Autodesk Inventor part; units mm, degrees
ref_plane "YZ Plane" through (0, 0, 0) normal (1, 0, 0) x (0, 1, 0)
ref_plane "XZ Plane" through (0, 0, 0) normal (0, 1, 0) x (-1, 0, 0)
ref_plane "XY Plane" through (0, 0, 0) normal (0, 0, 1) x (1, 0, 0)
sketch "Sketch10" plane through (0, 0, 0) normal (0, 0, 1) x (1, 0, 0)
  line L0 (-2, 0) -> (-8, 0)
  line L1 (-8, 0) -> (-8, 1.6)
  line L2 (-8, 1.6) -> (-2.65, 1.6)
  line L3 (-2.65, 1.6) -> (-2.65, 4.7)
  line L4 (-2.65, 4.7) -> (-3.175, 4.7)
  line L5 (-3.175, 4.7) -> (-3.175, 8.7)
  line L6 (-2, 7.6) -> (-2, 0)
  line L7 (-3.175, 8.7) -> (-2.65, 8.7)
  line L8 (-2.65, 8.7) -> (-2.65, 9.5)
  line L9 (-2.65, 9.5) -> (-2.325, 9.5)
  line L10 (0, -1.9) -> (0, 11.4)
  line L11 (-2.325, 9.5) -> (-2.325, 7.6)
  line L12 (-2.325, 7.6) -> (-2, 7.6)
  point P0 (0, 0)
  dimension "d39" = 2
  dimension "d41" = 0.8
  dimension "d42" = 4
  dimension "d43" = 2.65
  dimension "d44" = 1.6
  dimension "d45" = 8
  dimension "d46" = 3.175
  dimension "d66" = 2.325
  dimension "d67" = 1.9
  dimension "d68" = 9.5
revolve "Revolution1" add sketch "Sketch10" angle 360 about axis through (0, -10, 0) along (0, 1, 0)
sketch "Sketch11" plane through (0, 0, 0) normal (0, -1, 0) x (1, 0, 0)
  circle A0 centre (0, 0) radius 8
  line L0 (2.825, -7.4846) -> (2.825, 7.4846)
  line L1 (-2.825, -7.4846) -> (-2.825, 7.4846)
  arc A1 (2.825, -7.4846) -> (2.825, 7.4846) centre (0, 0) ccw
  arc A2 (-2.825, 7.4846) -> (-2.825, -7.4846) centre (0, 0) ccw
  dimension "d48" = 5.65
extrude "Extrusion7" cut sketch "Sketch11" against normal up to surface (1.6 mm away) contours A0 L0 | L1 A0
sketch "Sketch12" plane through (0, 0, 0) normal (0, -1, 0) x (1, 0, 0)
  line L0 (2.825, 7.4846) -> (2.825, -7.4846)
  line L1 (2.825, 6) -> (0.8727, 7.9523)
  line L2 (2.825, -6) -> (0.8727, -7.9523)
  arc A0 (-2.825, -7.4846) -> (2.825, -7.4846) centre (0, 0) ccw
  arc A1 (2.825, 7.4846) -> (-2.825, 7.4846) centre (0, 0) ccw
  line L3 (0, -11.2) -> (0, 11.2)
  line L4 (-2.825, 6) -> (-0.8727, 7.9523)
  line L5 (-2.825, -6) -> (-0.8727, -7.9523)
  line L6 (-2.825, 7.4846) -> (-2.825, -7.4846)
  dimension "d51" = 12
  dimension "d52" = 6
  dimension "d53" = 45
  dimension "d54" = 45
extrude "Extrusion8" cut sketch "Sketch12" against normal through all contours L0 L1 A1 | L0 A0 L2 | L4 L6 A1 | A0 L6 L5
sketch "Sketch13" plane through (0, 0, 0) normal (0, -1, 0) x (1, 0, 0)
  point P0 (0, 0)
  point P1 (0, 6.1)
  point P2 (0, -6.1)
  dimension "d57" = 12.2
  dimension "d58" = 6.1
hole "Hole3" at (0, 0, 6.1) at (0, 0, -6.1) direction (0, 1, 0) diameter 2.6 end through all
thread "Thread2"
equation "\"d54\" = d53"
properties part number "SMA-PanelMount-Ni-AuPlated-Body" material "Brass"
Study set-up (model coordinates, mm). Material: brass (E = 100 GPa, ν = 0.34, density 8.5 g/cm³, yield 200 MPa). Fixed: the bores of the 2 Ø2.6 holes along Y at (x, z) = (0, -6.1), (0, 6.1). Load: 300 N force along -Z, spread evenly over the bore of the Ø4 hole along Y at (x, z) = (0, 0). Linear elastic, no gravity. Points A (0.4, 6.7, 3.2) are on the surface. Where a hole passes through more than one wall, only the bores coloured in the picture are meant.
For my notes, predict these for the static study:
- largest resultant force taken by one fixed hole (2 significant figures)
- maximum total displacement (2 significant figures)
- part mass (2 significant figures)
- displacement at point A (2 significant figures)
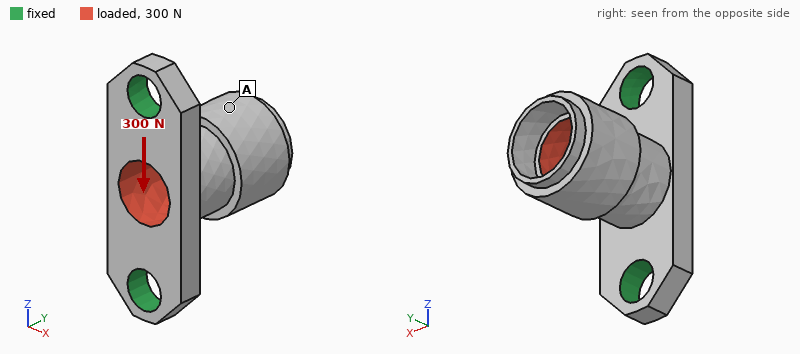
190 N
18 µm
1.7 g
14 µm
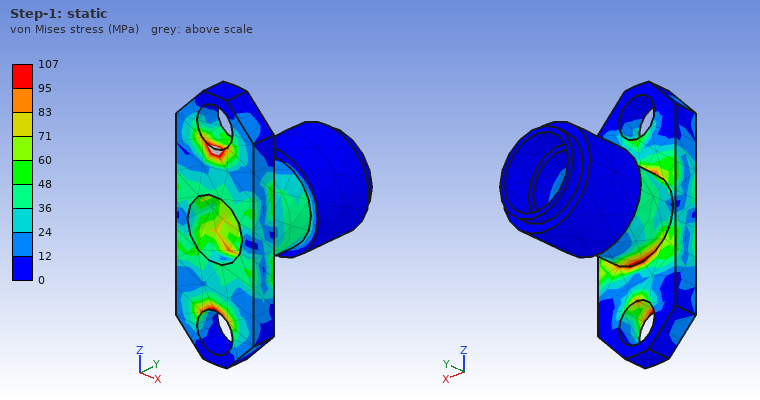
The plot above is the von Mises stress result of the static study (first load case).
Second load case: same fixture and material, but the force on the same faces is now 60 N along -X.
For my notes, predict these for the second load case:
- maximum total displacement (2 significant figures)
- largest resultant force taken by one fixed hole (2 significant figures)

12 µm
30 N
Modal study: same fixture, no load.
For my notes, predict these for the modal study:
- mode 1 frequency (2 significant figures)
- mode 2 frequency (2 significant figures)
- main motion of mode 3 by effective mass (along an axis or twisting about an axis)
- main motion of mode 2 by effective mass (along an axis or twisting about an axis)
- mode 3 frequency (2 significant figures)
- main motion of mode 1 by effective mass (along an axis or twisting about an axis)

11 kHz
19 kHz
along Y
along Z
30 kHz
along X
